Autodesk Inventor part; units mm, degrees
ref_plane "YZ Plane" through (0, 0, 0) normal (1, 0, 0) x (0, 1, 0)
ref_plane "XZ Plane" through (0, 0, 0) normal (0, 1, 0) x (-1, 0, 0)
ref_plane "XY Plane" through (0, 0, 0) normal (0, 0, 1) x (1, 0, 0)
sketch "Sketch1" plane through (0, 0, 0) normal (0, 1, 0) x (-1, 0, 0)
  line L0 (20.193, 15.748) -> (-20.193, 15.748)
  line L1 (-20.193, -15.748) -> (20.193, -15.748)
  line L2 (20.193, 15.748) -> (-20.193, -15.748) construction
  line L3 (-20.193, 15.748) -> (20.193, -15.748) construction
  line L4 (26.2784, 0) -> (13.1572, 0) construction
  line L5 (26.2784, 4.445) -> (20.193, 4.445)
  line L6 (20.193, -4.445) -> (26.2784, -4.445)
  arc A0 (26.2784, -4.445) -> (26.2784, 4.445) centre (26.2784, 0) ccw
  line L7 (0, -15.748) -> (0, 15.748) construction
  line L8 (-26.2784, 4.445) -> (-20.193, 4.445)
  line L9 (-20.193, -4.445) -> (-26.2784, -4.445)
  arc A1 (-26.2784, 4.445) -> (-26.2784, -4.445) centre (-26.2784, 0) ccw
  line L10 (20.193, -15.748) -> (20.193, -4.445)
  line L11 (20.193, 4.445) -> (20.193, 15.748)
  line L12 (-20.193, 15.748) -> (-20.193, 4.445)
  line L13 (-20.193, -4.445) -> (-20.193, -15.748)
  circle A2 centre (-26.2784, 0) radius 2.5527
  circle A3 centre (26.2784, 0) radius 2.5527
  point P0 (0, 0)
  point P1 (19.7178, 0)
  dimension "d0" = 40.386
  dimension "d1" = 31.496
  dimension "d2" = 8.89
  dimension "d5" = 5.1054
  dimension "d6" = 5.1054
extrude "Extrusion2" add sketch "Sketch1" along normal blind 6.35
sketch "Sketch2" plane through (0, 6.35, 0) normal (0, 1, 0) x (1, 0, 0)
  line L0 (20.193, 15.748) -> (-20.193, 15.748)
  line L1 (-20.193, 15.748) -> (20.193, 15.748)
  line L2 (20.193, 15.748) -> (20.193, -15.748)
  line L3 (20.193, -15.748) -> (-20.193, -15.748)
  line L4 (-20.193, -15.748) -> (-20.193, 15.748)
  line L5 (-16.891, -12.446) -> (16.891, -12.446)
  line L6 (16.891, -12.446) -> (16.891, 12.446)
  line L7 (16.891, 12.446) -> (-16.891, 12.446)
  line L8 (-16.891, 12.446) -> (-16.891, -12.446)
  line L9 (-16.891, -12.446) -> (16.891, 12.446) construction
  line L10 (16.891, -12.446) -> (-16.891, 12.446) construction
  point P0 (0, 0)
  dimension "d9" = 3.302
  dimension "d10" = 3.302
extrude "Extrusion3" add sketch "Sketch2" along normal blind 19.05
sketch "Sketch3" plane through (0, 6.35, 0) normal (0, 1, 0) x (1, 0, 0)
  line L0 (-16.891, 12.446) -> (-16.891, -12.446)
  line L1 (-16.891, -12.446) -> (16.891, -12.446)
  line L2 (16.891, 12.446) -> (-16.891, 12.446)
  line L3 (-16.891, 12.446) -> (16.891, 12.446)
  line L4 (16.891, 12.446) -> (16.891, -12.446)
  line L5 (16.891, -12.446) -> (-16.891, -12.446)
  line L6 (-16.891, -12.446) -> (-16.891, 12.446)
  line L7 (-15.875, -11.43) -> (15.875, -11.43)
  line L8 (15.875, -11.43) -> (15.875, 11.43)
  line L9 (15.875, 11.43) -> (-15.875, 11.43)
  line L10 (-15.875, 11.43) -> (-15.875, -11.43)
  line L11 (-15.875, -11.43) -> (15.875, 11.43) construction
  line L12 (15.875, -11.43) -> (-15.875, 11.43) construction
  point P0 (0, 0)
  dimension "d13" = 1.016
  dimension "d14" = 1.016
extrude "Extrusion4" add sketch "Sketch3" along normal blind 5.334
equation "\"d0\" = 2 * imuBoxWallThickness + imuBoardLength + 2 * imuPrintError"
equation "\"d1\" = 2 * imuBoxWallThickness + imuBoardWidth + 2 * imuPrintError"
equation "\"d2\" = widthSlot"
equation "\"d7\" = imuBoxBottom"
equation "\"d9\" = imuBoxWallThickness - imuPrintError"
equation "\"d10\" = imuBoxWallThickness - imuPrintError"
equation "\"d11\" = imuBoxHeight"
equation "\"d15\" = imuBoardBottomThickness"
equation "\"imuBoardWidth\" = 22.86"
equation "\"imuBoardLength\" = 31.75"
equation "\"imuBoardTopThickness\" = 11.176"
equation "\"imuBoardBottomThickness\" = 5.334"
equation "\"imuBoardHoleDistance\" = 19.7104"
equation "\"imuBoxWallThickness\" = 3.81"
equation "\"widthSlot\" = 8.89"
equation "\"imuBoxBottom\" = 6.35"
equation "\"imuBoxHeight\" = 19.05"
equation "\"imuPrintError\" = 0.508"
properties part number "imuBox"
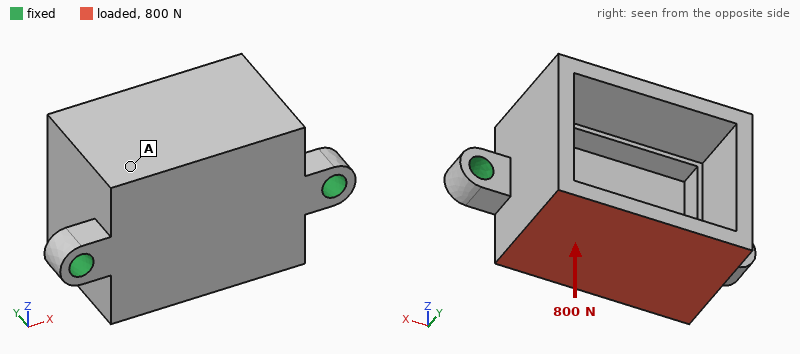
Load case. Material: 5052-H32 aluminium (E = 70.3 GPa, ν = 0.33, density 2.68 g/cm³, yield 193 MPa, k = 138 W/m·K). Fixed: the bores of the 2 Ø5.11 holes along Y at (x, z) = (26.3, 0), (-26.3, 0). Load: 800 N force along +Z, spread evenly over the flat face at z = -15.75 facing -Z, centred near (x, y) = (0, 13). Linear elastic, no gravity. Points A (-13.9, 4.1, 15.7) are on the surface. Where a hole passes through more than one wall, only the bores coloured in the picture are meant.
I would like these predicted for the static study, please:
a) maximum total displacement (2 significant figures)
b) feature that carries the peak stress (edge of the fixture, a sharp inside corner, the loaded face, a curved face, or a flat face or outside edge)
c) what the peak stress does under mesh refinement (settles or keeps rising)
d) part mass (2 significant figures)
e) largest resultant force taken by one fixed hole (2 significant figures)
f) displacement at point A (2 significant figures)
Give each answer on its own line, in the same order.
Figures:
73 µm
edge of the fixture
keeps rising
48 g
400 N
29 µm
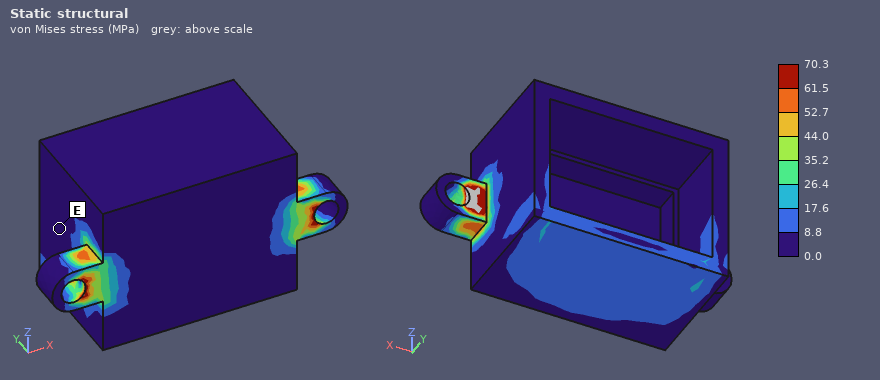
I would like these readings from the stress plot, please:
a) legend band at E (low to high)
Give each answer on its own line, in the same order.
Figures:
0.0 to 8.8 MPa
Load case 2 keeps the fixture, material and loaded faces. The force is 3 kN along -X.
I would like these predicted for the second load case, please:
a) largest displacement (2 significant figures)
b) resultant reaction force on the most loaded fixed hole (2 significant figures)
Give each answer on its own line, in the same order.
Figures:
46 µm
1.9 kN
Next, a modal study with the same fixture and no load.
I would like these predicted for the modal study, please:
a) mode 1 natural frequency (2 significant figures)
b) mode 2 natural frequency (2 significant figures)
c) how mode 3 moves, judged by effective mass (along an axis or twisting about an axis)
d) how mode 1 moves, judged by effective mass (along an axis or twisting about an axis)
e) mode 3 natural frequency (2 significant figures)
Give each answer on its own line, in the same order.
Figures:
3300 Hz
8300 Hz
along Y
along Z
9800 Hz
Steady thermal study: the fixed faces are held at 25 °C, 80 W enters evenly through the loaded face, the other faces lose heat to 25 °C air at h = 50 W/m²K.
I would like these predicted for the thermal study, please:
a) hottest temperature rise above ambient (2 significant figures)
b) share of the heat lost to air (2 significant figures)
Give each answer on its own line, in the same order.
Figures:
67 K
17 %
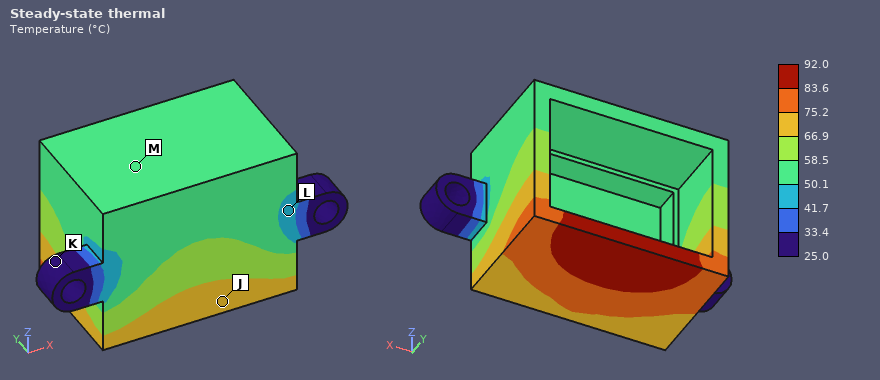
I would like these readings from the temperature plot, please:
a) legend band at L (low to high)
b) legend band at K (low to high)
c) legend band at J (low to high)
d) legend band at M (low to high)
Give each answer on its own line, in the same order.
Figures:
41.7 to 50.1 °C
25.0 to 33.4 °C
66.9 to 75.2 °C
50.1 to 58.5 °C
